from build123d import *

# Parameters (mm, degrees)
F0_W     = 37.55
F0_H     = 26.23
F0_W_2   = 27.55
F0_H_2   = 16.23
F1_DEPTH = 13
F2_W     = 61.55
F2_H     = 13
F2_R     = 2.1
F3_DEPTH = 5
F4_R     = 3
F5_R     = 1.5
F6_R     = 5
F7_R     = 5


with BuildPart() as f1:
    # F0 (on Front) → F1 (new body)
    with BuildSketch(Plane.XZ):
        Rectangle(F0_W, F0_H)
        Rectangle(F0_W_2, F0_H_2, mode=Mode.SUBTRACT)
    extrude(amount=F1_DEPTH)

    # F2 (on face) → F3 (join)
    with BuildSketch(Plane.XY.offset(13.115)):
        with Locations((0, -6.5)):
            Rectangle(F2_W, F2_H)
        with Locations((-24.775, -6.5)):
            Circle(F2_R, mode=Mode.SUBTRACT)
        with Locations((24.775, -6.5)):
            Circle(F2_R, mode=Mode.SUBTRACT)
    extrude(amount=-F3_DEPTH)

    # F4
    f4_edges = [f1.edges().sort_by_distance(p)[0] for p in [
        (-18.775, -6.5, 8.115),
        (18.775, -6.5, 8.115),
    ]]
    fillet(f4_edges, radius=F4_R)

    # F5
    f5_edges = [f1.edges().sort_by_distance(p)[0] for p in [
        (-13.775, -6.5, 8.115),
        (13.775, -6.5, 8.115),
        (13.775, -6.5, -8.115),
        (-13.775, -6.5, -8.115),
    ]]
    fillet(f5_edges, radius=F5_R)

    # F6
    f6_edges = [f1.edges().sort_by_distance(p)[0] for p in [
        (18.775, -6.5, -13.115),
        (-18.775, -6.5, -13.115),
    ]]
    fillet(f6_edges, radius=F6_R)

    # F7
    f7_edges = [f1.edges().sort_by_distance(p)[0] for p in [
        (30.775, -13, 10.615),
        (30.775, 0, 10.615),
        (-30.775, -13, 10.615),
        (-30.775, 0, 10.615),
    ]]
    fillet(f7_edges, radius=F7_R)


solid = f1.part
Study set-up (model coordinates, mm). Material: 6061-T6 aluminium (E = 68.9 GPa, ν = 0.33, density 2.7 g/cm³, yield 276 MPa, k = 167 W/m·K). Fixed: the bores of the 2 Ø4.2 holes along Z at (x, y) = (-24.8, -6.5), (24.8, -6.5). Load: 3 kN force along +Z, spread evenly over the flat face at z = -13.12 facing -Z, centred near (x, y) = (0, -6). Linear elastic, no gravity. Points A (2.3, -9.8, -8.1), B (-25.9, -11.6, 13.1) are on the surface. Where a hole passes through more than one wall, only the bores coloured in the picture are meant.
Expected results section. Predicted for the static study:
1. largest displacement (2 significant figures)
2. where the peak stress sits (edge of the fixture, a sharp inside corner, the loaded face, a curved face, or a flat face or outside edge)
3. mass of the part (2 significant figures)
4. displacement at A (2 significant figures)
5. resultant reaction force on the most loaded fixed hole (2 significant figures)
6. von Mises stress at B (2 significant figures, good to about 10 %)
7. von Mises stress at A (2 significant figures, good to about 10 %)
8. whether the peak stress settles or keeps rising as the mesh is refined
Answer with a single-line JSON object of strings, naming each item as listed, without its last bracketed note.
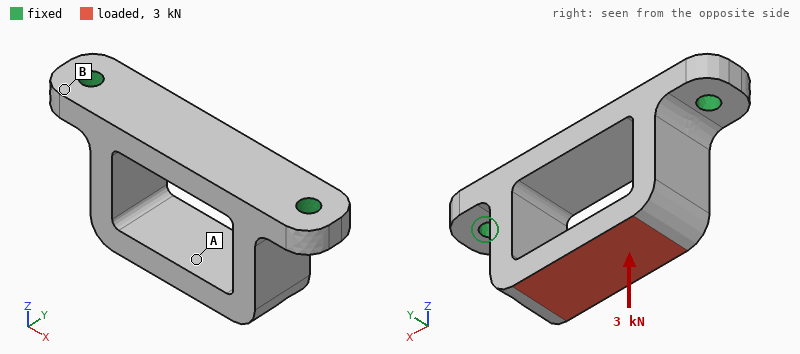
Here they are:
{"largest displacement": "72 µm", "where the peak stress sits": "edge of the fixture", "mass of the part": "22 g", "displacement at A": "67 µm", "resultant reaction force on the most loaded fixed hole": "1.6 kN", "von Mises stress at B": "22 MPa", "von Mises stress at A": "90 MPa", "whether the peak stress settles or keeps rising as the mesh is refined": "keeps rising"}
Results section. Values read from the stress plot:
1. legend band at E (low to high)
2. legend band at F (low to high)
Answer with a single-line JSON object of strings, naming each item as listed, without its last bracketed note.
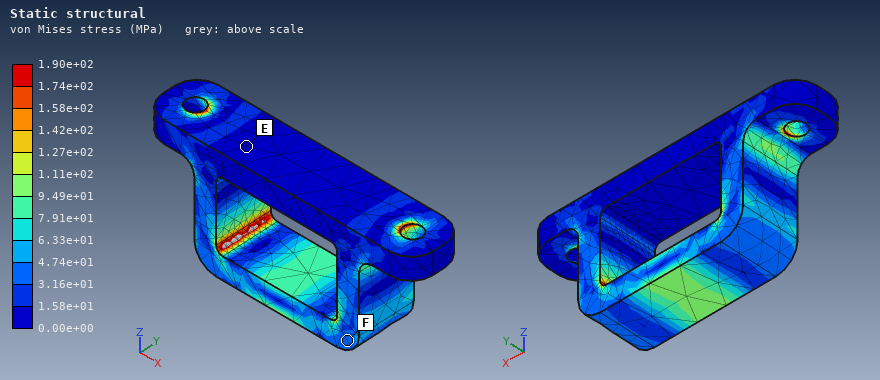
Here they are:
{"legend band at E": "0.00e+00 to 1.58e+01 MPa", "legend band at F": "3.16e+01 to 4.74e+01 MPa"}
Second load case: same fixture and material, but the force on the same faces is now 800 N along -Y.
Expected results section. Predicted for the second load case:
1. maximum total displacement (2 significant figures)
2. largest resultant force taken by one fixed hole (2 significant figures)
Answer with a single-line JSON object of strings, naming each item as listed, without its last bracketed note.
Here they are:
{"maximum total displacement": "0.14 mm", "largest resultant force taken by one fixed hole": "400 N"}
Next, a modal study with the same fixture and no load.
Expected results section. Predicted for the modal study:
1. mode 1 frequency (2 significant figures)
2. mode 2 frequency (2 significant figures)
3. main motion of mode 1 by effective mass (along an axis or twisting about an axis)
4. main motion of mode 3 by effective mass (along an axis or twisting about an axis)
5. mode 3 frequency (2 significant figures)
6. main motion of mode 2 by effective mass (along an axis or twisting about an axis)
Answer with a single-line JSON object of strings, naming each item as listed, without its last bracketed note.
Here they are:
{"mode 1 frequency": "4900 Hz", "mode 2 frequency": "7600 Hz", "main motion of mode 1 by effective mass": "along Y", "main motion of mode 3 by effective mass": "twisting about Z", "mode 3 frequency": "10 kHz", "main motion of mode 2 by effective mass": "along X"}
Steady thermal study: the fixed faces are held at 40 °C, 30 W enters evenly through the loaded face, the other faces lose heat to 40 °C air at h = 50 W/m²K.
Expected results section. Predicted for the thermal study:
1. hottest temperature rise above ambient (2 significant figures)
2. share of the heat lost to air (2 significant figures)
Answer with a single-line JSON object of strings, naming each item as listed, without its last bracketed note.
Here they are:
{"hottest temperature rise above ambient": "42 K", "share of the heat lost to air": "11 %"}
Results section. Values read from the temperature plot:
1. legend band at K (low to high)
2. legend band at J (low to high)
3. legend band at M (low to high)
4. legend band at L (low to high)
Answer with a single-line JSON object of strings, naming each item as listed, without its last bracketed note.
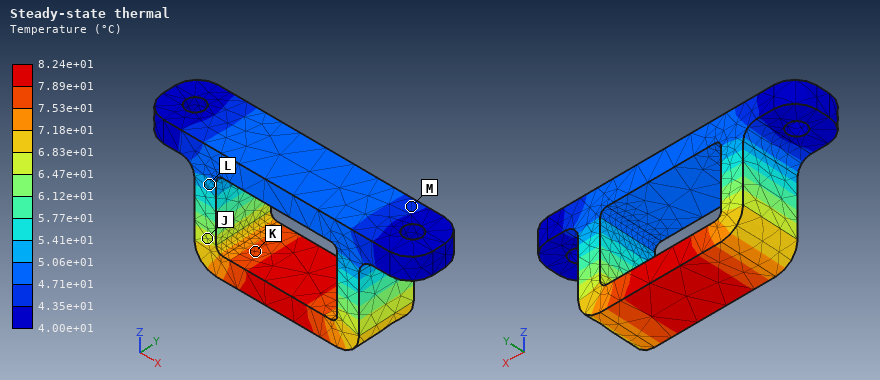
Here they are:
{"legend band at K": "7.53e+01 to 7.89e+01 °C", "legend band at J": "6.47e+01 to 6.83e+01 °C", "legend band at M": "4.35e+01 to 4.71e+01 °C", "legend band at L": "5.06e+01 to 5.41e+01 °C"}
